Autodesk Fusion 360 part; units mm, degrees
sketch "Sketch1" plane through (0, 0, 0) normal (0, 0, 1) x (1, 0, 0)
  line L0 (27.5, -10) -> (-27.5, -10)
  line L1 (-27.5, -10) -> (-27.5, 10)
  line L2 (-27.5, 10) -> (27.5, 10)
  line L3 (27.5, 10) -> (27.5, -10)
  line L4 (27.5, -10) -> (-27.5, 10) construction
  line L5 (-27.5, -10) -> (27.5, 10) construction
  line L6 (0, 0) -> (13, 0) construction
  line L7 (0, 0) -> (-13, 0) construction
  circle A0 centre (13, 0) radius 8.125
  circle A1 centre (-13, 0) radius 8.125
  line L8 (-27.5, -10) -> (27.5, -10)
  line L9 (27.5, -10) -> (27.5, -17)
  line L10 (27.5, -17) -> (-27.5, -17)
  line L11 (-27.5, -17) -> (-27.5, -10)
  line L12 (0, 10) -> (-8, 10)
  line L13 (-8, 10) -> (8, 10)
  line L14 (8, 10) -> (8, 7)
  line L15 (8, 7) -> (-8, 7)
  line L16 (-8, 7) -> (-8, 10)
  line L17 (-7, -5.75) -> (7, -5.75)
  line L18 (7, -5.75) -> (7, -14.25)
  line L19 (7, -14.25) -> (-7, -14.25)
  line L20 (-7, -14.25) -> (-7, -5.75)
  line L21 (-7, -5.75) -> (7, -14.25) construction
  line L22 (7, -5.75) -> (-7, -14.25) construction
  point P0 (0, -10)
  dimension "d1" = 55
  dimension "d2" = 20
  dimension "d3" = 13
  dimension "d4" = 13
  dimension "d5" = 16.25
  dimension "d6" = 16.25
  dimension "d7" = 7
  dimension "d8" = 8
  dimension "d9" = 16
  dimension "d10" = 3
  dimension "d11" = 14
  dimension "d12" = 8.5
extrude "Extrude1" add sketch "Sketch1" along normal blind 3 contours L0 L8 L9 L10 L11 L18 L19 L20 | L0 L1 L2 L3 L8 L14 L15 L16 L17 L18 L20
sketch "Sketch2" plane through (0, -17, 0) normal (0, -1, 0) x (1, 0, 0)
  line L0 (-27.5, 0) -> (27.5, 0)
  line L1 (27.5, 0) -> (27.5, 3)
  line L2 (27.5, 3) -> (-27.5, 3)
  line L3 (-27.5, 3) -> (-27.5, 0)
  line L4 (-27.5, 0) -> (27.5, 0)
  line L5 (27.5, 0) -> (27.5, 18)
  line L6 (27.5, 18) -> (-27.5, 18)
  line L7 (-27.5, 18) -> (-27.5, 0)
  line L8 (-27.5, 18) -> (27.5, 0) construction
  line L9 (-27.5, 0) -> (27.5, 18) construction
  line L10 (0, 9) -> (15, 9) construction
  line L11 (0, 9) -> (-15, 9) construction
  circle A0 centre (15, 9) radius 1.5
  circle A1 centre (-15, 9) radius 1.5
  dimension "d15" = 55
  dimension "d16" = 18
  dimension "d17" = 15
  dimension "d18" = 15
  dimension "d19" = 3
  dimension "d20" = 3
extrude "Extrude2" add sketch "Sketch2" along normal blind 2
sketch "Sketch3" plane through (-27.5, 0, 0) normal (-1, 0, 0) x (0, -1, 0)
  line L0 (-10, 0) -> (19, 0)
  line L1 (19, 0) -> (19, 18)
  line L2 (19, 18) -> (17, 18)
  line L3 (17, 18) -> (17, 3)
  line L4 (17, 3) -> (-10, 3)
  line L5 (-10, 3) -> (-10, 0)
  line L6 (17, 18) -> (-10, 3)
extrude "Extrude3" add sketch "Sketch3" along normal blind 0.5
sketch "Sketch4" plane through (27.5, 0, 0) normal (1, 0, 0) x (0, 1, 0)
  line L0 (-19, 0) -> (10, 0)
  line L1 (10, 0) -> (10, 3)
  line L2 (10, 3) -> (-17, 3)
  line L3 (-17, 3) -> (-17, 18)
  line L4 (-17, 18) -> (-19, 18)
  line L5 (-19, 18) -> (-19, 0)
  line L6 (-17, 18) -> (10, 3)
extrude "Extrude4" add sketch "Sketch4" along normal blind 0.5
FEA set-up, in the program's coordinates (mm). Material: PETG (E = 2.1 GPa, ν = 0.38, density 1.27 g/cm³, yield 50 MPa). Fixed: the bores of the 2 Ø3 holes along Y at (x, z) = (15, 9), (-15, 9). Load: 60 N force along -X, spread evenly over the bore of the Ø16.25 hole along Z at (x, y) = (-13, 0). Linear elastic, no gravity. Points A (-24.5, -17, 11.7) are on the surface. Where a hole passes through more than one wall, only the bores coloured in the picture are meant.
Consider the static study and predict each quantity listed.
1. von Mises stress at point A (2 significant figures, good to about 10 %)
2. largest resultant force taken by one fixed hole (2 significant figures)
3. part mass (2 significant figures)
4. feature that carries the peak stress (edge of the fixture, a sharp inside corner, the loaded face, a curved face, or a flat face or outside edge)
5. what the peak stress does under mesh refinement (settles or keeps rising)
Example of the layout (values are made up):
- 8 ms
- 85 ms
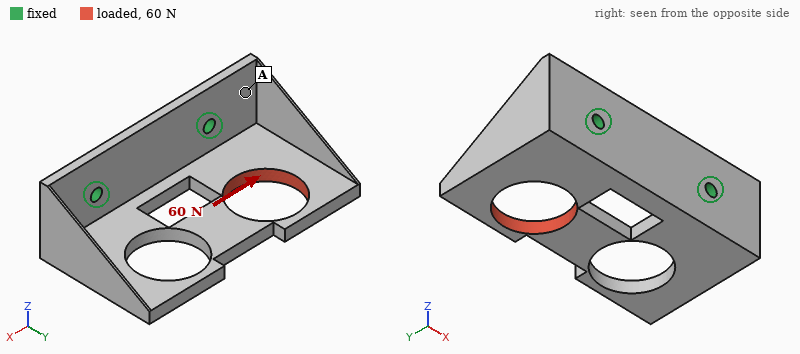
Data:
- 3.0 MPa
- 47 N
- 6.3 g
- a sharp inside corner
- keeps rising
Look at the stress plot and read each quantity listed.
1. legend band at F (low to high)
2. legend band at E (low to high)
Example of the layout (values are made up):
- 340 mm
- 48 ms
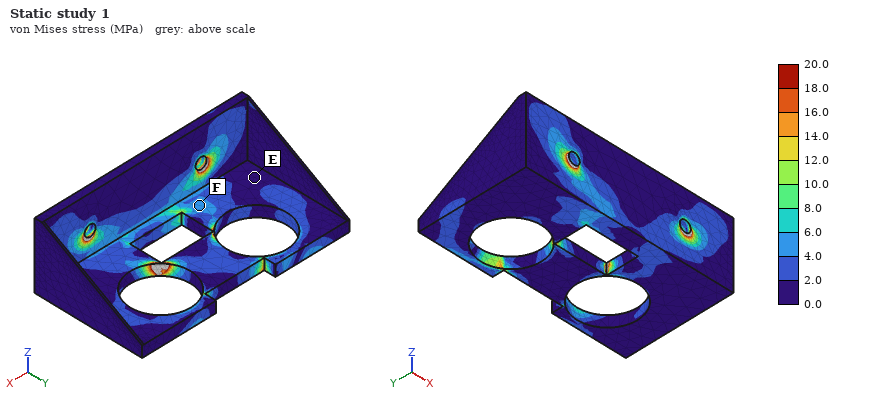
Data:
- 4.0 to 6.0 MPa
- 0.0 to 2.0 MPa
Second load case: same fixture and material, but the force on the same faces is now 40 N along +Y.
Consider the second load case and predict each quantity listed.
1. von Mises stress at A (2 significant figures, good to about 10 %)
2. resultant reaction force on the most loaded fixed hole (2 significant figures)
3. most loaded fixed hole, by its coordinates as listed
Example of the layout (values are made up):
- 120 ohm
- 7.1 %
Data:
- 3.5 MPa
- 36 N
- (-15, 9)
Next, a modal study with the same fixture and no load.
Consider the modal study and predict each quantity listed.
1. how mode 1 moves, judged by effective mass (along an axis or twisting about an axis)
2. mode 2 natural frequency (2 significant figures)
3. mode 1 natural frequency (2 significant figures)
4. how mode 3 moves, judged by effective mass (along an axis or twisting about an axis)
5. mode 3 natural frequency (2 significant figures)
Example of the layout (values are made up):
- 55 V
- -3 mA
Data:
- along Z
- 700 Hz
- 510 Hz
- along X
- 1500 Hz
